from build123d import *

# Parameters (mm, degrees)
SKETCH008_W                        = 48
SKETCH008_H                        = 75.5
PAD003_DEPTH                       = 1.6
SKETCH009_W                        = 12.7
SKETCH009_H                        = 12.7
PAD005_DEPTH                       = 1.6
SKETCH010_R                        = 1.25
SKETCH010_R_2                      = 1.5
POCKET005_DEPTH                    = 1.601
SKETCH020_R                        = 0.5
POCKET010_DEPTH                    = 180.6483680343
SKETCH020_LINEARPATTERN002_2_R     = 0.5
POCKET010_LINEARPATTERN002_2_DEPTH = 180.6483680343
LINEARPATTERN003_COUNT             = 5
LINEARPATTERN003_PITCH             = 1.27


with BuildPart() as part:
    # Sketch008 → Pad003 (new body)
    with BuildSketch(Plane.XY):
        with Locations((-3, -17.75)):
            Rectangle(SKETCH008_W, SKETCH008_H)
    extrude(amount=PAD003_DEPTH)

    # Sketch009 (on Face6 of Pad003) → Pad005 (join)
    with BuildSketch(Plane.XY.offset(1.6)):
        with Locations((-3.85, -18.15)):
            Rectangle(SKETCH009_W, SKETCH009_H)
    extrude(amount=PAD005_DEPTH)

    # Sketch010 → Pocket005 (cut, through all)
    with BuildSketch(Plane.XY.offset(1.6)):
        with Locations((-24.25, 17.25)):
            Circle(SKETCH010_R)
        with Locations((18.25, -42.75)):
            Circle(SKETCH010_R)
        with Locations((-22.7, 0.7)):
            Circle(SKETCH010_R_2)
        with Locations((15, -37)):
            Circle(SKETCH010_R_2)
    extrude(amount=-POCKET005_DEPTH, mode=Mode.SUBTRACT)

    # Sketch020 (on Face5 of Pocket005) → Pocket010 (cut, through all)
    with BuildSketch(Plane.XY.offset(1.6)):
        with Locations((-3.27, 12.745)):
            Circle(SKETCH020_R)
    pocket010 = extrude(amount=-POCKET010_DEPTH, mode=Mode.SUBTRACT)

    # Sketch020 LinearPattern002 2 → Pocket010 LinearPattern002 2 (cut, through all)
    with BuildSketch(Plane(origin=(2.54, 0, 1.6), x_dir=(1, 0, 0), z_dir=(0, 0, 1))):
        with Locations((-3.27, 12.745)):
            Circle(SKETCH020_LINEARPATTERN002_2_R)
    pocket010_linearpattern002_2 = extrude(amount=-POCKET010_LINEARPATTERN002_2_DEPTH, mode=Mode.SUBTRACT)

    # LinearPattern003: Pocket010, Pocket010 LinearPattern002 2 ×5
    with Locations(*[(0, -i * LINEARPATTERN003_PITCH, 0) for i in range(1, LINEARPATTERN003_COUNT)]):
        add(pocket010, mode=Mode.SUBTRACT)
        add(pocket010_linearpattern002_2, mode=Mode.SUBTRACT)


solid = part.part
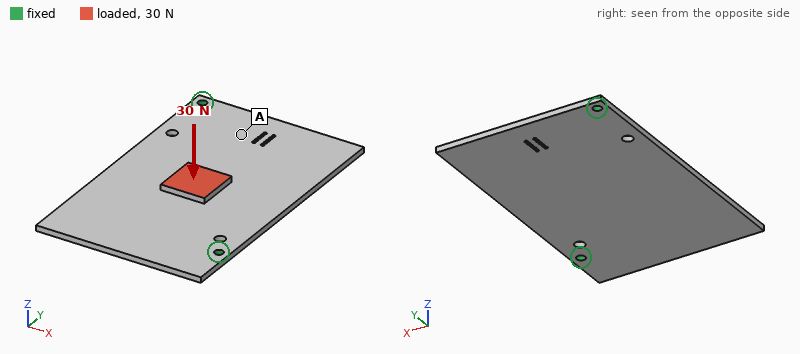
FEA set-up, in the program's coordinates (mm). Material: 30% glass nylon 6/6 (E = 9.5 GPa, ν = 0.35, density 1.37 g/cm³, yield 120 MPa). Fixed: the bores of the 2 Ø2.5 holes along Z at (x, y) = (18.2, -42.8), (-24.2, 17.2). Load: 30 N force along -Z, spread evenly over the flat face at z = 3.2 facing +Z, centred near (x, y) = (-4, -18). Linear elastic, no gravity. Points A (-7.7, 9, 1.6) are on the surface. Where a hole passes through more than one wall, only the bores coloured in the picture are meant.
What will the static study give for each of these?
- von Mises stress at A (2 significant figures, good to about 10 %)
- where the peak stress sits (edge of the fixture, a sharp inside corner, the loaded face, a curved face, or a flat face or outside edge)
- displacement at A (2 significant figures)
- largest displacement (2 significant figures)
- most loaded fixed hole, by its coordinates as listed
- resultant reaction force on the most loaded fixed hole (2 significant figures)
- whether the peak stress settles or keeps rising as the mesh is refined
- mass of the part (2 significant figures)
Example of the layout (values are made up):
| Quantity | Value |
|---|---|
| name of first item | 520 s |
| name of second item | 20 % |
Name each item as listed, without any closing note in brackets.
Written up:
| Quantity | Value |
|---|---|
| von Mises stress at A | 4.4 MPa |
| where the peak stress sits | edge of the fixture |
| displacement at A | 0.22 mm |
| largest displacement | 0.83 mm |
| most loaded fixed hole, by its coordinates as listed | (18.2, -42.8) |
| resultant reaction force on the most loaded fixed hole | 19 N |
| whether the peak stress settles or keeps rising as the mesh is refined | keeps rising |
| mass of the part | 8.2 g |
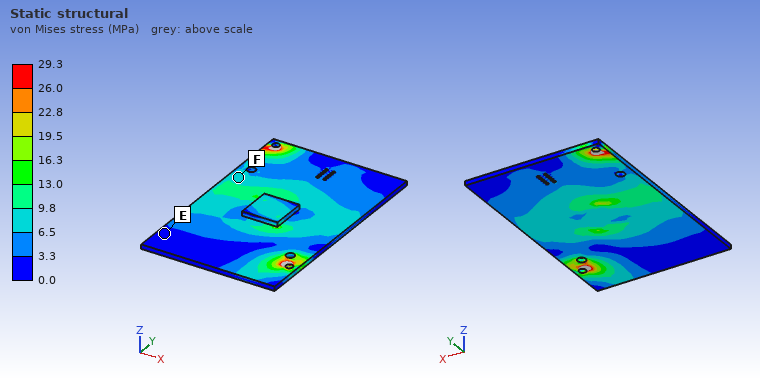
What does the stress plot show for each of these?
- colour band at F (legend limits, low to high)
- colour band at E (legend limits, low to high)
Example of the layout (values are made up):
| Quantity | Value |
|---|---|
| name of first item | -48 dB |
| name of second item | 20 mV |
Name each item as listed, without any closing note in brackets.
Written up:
| Quantity | Value |
|---|---|
| colour band at F | 6.5 to 9.8 MPa |
| colour band at E | 0.0 to 3.3 MPa |
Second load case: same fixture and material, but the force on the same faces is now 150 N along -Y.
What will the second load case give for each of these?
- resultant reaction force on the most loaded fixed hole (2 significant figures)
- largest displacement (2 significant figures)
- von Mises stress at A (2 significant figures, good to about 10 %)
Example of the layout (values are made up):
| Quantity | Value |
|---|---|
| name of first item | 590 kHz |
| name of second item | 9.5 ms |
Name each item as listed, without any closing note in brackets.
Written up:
| Quantity | Value |
|---|---|
| resultant reaction force on the most loaded fixed hole | 76 N |
| largest displacement | 0.83 mm |
| von Mises stress at A | 3.7 MPa |
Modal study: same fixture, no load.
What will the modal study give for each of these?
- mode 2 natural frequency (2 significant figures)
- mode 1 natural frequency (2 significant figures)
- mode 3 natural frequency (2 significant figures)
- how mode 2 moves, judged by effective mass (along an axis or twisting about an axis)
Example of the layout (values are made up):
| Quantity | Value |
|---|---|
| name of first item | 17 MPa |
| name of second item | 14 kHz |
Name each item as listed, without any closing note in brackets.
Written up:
| Quantity | Value |
|---|---|
| mode 2 natural frequency | 490 Hz |
| mode 1 natural frequency | 340 Hz |
| mode 3 natural frequency | 1000 Hz |
| how mode 2 moves, judged by effective mass | along Z |
